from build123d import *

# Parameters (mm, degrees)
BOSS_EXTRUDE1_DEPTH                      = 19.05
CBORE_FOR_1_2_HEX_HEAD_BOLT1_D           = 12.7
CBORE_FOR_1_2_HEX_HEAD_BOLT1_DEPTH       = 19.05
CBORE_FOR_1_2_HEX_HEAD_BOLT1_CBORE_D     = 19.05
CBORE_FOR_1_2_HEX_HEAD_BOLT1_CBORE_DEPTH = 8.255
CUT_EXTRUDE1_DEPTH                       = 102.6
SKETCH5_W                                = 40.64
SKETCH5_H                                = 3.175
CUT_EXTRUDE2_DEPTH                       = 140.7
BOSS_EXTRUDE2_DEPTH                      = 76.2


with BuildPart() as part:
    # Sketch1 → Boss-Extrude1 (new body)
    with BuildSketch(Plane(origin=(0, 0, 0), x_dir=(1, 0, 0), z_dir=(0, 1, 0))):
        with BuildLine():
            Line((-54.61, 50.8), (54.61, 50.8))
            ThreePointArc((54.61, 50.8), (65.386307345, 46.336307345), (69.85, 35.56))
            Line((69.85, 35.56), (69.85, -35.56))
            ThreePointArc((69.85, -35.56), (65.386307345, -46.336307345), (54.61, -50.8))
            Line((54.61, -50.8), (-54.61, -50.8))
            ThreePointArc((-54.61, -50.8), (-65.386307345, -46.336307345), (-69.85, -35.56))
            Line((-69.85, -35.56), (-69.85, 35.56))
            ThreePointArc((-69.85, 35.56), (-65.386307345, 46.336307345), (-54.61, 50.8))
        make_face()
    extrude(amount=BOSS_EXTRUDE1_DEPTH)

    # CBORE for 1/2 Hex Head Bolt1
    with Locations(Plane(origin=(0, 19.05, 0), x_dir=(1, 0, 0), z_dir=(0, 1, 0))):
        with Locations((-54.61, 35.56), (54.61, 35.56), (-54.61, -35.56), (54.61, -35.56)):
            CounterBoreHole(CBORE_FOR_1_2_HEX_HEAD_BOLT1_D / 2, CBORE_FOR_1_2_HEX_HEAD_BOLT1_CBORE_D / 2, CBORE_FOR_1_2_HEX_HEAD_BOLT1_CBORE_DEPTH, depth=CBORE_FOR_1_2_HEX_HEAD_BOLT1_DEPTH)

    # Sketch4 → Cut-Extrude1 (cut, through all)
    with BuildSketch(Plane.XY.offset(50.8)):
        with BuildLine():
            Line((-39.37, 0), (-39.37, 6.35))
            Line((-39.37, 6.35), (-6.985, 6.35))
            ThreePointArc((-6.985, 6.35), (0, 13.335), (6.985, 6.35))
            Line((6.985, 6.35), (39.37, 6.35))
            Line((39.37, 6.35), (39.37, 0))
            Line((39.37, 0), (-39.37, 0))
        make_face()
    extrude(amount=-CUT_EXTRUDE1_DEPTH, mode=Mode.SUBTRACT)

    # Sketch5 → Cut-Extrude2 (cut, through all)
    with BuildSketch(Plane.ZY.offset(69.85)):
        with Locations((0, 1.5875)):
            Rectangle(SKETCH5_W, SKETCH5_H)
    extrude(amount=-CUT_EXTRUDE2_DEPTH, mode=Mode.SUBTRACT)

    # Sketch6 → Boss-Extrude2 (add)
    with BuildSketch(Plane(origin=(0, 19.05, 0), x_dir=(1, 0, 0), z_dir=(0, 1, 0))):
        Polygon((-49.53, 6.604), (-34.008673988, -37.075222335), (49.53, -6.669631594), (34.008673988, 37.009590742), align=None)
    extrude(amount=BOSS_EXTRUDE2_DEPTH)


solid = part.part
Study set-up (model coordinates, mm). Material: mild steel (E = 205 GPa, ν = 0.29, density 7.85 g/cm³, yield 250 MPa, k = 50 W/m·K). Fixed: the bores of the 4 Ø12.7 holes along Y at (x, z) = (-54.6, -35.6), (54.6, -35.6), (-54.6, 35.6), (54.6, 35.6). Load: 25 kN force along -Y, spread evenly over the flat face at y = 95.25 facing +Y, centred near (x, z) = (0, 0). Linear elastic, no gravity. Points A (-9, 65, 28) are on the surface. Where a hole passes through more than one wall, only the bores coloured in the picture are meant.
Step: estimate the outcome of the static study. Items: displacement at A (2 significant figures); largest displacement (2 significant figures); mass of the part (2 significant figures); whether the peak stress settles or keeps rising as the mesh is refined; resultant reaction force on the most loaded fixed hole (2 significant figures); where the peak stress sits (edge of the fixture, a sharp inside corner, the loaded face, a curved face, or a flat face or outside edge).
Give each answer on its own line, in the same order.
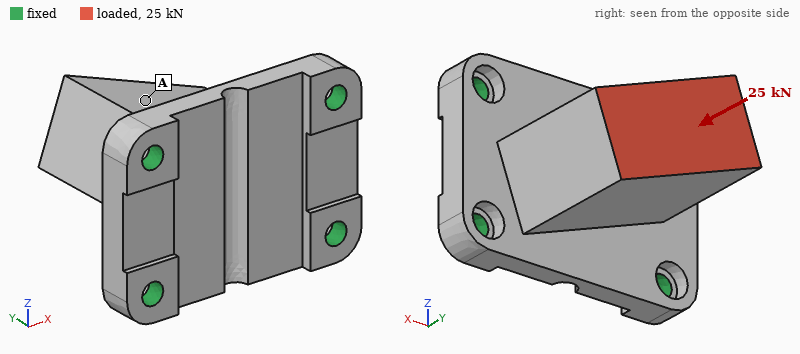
11 µm
12 µm
3.9 kg
keeps rising
11 kN
edge of the fixture
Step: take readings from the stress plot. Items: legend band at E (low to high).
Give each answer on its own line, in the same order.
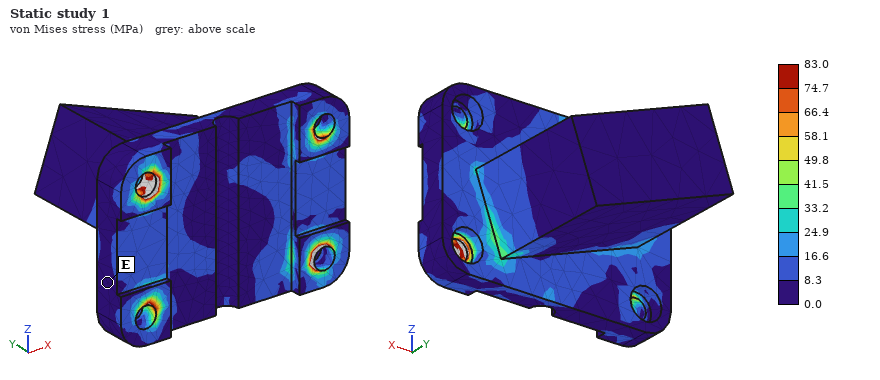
0.0 to 8.3 MPa
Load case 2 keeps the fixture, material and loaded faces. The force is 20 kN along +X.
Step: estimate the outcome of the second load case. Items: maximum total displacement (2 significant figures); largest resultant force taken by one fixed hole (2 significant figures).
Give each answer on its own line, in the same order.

52 µm
12 kN
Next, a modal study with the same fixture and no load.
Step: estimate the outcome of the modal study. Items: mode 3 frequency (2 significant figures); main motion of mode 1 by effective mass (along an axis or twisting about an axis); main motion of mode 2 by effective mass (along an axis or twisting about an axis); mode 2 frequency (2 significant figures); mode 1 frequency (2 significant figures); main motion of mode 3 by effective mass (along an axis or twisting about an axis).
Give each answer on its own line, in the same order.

4500 Hz
along Z
along X
3800 Hz
2300 Hz
along Y
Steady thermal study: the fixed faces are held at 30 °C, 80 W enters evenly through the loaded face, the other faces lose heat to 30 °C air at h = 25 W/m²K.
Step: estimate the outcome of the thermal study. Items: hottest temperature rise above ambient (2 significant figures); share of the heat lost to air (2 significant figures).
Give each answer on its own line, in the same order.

44 K
28 %
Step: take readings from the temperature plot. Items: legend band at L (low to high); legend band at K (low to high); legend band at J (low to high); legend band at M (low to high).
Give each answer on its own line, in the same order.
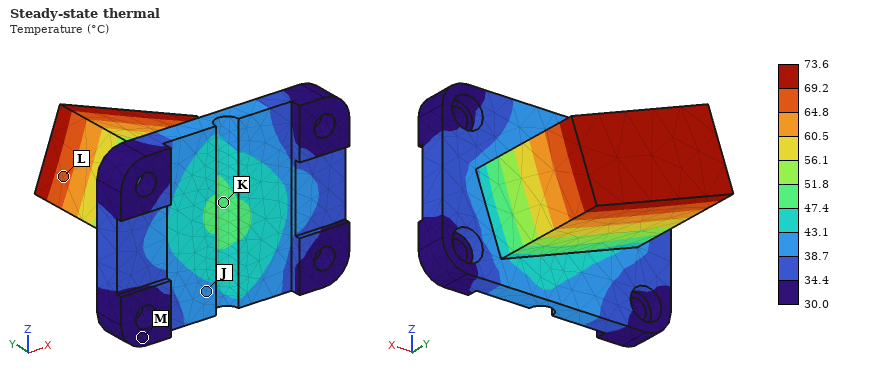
64.8 to 69.2 °C
47.4 to 51.8 °C
38.7 to 43.1 °C
30.0 to 34.4 °C
